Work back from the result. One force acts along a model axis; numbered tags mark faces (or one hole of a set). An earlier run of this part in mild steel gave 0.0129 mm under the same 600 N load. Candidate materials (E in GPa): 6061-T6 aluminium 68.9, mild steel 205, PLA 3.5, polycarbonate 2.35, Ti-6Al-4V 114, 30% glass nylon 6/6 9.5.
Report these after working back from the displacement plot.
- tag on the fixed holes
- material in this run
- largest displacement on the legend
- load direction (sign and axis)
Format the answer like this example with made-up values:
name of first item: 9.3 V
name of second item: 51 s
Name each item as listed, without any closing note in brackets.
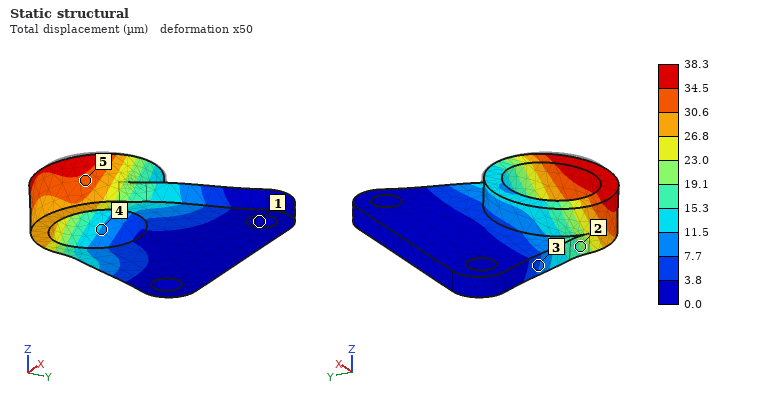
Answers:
tag on the fixed holes: 1
material in this run: 6061-T6 aluminium
largest displacement on the legend: 38.3 µm
load direction: -X
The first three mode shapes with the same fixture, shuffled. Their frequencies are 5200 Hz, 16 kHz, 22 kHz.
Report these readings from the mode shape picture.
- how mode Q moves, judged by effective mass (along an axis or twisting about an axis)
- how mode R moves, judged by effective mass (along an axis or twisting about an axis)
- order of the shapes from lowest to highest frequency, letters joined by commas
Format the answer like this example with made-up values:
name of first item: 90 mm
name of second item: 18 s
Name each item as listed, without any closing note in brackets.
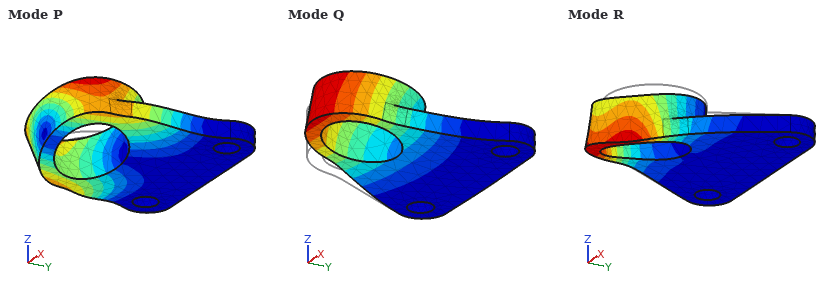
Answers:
how mode Q moves, judged by effective mass: along Z
how mode R moves, judged by effective mass: along X
order of the shapes from lowest to highest frequency, letters joined by commas: Q, P, R
